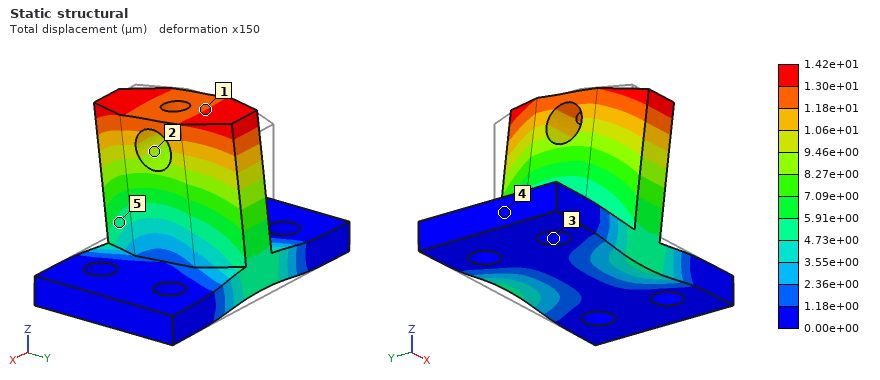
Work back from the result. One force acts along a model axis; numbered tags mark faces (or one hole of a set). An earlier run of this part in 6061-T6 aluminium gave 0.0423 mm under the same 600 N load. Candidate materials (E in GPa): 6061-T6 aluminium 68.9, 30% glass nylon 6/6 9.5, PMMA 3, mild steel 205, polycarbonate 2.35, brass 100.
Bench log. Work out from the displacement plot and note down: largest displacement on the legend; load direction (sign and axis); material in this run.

1.42e+01 µm
-Y
mild steel
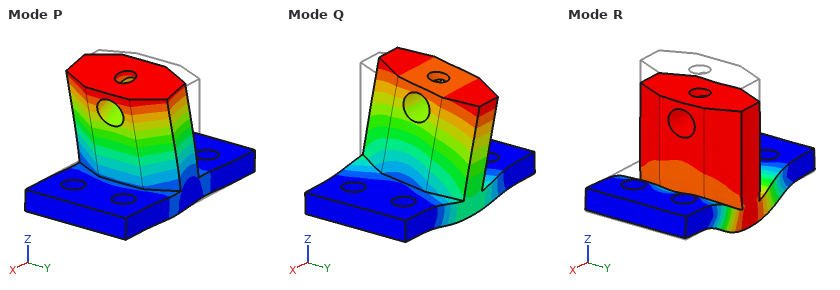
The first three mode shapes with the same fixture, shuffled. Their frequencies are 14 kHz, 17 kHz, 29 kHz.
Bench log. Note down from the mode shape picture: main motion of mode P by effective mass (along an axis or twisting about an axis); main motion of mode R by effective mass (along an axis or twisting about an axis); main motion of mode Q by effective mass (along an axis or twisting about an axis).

along X
along Z
along Y
